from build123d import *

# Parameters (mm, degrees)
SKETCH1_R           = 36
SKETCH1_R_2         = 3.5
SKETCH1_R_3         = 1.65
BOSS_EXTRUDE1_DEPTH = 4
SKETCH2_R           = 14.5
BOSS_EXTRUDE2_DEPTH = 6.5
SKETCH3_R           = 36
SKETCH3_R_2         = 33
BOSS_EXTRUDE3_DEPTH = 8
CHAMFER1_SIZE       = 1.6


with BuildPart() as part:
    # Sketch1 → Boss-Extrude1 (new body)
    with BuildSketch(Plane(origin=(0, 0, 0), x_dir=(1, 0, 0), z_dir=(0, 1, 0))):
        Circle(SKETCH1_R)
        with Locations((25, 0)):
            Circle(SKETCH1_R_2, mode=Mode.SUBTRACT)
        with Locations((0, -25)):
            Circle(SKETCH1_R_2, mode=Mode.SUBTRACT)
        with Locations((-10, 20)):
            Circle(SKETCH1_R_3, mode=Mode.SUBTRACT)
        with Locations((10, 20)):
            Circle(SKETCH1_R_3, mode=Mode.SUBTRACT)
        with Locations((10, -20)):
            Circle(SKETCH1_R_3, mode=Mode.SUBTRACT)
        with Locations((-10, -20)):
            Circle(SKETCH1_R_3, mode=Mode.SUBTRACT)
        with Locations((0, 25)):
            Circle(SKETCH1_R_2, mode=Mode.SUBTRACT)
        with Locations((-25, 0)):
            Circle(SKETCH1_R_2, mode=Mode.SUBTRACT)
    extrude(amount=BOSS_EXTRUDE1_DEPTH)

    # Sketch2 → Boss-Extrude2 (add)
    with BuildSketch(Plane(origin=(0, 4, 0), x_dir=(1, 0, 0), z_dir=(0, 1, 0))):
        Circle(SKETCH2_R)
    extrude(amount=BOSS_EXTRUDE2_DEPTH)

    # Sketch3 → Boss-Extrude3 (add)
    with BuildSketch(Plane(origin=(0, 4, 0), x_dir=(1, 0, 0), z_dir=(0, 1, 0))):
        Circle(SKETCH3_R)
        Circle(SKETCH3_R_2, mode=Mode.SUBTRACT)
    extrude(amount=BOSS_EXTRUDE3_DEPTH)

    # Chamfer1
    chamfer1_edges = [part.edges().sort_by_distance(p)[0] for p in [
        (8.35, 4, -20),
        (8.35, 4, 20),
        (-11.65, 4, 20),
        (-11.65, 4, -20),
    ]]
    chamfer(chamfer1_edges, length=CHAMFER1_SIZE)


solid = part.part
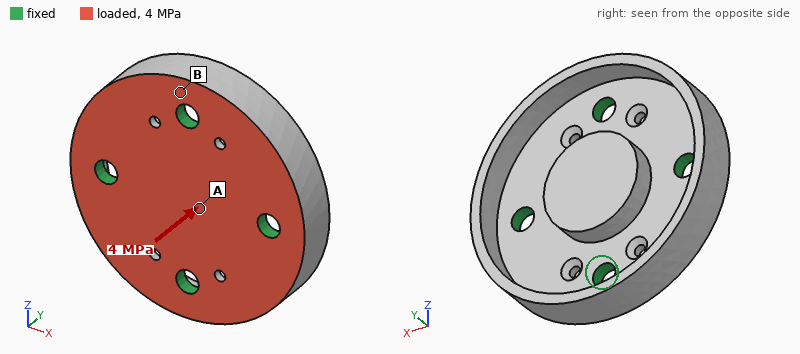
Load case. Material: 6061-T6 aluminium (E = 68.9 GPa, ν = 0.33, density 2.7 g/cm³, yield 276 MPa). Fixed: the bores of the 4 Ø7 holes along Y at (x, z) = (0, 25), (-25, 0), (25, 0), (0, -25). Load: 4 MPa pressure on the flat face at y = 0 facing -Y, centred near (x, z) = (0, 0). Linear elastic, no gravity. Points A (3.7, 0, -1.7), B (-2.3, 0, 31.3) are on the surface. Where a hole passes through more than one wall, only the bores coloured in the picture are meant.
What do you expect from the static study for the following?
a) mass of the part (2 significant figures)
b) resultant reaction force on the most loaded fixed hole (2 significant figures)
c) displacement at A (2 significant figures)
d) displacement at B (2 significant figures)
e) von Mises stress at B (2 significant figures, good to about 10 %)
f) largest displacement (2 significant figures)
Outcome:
67 g
3.9 kN
28 µm
8.4 µm
53 MPa
39 µm
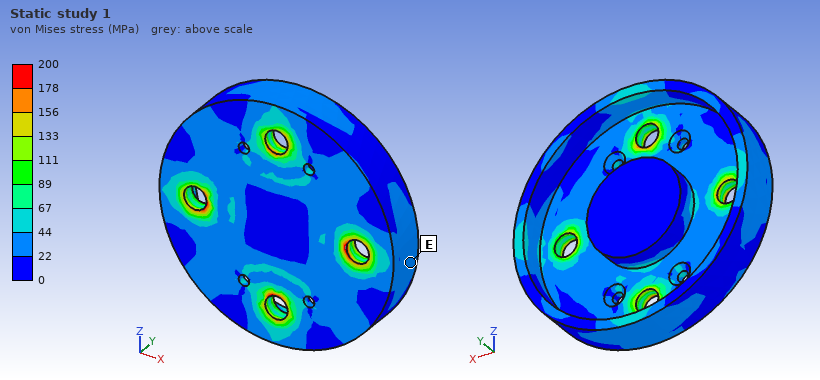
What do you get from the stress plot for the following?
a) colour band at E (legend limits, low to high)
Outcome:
22 to 44 MPa
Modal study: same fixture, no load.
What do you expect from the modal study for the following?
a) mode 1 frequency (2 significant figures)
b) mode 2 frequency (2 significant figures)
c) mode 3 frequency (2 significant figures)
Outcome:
8100 Hz
11 kHz
11 kHz
